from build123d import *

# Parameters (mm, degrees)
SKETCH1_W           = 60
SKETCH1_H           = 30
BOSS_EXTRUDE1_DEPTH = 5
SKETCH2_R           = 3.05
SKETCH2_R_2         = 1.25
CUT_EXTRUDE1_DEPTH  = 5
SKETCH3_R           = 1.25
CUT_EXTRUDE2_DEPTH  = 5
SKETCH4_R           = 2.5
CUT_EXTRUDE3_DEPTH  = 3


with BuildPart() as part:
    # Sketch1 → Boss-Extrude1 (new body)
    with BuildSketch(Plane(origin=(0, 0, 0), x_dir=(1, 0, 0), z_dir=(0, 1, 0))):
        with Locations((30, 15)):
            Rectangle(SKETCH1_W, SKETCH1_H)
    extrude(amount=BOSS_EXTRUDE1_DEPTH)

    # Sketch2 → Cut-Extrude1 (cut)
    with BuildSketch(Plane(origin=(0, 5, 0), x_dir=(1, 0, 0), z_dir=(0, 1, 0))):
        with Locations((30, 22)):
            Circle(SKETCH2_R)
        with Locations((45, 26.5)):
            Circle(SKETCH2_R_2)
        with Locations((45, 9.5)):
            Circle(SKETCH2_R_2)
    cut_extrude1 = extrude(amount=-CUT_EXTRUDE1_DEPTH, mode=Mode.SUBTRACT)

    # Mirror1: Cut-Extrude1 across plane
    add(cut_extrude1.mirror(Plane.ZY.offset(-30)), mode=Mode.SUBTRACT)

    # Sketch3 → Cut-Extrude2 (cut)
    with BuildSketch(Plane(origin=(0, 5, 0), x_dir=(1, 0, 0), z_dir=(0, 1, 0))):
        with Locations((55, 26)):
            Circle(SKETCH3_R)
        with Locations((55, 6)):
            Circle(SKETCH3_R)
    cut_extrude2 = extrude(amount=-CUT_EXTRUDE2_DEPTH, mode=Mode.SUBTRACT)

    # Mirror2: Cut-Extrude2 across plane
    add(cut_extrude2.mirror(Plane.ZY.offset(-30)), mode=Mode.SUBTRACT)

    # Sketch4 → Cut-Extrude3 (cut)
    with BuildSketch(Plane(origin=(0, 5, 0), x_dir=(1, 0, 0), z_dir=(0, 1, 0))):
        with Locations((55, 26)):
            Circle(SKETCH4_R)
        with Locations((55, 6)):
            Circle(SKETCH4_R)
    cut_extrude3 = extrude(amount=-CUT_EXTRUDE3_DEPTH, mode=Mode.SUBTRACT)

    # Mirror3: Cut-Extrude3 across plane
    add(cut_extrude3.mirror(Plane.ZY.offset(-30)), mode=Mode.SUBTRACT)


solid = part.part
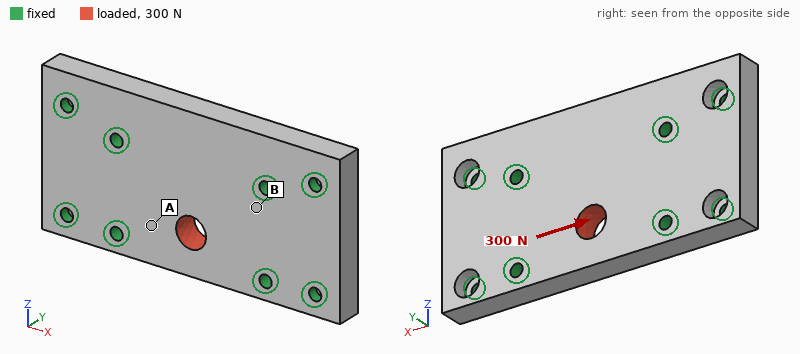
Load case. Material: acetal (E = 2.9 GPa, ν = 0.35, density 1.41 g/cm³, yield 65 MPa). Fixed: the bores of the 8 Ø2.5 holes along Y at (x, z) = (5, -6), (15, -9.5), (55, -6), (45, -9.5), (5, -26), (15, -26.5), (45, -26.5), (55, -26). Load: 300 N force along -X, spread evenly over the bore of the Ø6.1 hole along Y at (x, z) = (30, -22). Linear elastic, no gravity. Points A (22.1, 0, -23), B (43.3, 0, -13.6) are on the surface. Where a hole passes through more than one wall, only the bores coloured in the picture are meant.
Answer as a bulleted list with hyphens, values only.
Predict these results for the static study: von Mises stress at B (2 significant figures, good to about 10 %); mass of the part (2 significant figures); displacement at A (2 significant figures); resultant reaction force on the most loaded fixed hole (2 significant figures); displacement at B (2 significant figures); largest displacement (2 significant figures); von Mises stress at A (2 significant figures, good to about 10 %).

- 1.1 MPa
- 12 g
- 6.1 µm
- 87 N
- 2.2 µm
- 12 µm
- 2.4 MPa
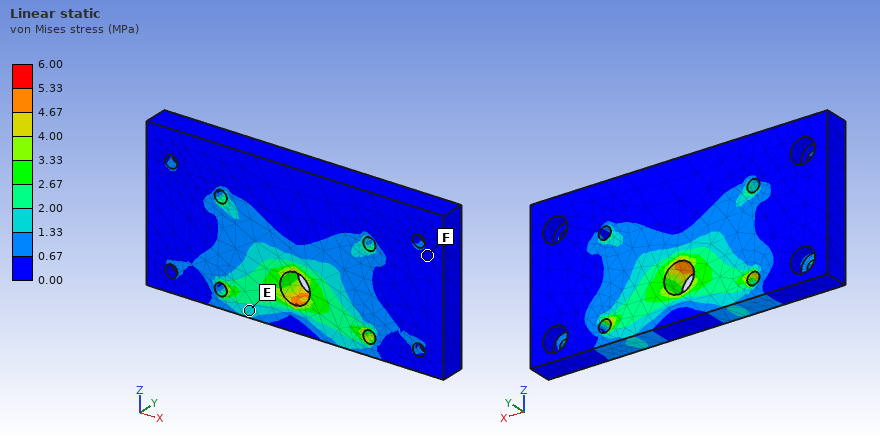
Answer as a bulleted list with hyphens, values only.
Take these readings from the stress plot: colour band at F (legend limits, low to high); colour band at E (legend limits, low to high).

- 0.00 to 0.67 MPa
- 1.33 to 2.00 MPa
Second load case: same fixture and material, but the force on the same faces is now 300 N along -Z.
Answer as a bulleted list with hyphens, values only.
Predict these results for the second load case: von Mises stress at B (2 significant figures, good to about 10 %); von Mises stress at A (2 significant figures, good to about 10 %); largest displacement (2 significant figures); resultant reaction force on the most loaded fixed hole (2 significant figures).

- 2.3 MPa
- 2.5 MPa
- 27 µm
- 96 N
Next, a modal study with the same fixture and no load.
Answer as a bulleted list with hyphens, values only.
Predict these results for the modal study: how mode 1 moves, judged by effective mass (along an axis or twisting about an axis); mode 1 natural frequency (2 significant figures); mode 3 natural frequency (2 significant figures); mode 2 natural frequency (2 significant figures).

- along Y
- 6000 Hz
- 10 kHz
- 7300 Hz
